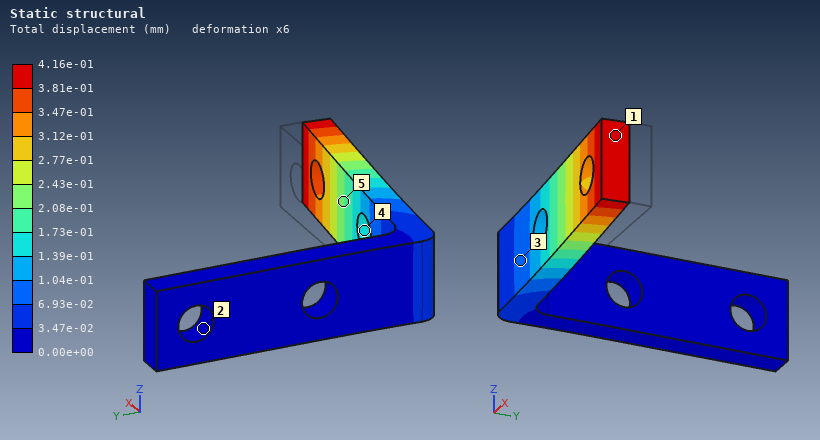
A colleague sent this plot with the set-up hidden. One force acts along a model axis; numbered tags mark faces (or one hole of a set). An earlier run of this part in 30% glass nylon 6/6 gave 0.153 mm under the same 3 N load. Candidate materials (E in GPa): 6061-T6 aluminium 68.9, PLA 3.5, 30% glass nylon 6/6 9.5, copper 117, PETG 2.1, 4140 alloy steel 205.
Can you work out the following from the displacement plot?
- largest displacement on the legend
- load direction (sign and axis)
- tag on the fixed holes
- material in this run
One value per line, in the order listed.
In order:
4.16e-01 mm
-Y
2
PLA
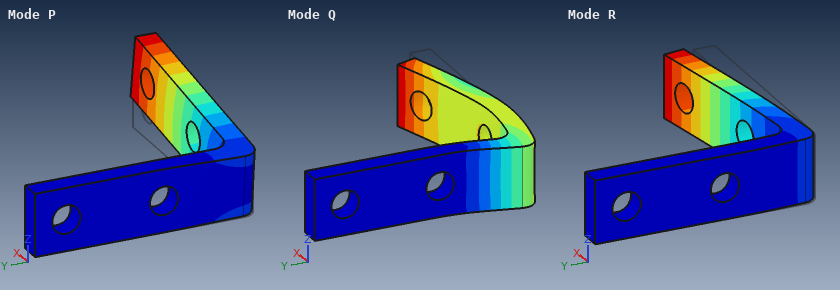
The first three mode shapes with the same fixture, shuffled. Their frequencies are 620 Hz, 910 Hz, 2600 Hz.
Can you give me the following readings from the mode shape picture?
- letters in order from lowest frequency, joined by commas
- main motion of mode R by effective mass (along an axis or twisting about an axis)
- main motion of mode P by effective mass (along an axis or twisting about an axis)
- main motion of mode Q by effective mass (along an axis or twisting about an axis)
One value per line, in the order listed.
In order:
R, P, Q
along Y
along Z
along X
